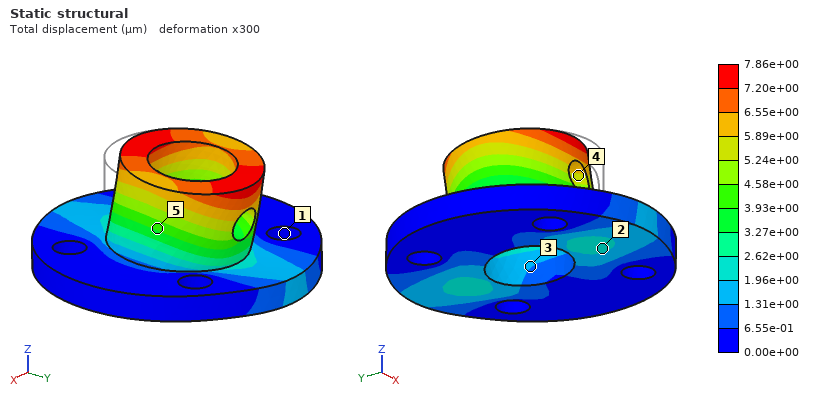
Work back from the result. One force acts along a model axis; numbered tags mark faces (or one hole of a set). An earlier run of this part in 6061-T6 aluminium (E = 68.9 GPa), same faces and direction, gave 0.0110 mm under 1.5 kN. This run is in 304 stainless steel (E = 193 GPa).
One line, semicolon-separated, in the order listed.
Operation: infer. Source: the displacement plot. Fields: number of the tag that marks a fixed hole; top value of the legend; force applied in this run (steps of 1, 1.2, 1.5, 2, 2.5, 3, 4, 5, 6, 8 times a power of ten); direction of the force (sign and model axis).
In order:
1; 7.86e+00 µm; 3 kN; +Y
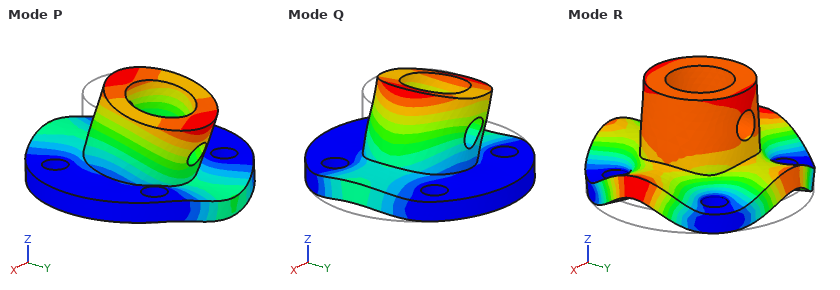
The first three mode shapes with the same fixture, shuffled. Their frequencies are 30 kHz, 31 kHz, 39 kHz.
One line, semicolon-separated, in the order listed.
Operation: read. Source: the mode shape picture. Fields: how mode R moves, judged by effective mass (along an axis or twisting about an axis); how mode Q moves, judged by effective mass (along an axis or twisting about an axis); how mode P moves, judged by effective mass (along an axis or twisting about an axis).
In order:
along Z; along X; along Y
